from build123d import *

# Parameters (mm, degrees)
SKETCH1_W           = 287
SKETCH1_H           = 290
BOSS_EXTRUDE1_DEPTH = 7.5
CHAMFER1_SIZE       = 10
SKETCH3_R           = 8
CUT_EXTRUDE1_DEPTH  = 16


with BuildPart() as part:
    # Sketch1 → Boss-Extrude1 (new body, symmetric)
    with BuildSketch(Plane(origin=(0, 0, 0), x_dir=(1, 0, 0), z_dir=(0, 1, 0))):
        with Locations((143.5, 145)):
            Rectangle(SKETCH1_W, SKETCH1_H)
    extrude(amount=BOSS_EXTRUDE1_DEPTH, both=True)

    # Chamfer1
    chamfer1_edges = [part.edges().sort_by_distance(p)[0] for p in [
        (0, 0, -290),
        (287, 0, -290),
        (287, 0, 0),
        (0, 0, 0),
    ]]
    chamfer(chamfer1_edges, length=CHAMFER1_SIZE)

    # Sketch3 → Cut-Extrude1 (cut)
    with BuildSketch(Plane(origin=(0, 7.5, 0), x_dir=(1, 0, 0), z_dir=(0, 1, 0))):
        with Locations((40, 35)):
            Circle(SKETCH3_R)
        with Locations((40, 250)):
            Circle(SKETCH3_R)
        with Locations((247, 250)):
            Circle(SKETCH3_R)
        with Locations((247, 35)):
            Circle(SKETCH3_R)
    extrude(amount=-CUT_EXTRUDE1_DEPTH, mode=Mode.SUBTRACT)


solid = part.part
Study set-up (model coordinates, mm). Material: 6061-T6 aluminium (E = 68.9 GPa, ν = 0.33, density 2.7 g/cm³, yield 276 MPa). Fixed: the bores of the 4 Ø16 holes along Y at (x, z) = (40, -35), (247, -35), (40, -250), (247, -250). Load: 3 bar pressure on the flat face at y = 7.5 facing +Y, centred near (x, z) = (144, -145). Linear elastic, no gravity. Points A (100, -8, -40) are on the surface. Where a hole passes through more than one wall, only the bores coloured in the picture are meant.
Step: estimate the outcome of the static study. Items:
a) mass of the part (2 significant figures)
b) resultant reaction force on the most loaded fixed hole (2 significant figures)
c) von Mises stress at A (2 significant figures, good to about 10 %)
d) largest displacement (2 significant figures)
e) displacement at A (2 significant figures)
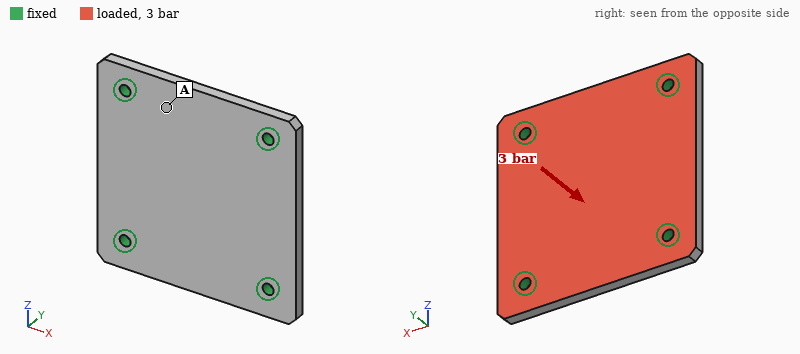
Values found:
3.3 kg
6.3 kN
11 MPa
0.19 mm
0.076 mm
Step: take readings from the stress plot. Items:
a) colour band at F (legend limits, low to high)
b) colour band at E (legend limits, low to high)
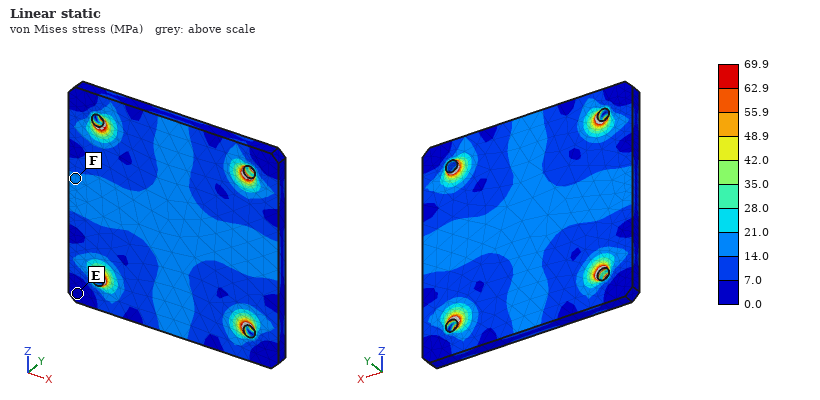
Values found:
14.0 to 21.0 MPa
0.0 to 7.0 MPa
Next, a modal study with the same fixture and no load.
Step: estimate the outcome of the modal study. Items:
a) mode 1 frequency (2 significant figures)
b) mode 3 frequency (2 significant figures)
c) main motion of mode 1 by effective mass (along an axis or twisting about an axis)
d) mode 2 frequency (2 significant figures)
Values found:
1200 Hz
1800 Hz
along Y
1800 Hz
